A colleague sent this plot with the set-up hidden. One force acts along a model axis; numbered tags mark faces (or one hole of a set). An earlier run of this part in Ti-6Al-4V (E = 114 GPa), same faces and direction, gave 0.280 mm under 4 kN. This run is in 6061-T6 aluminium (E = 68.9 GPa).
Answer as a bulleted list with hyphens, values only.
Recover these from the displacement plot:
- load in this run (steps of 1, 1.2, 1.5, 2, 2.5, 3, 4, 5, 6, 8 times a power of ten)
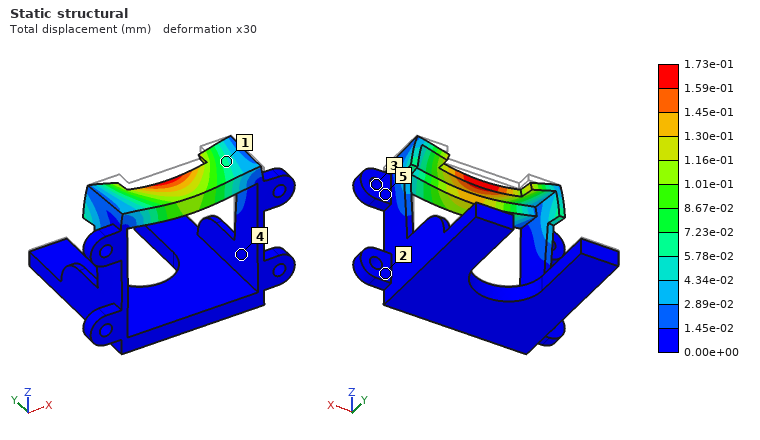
- 1.5 kN
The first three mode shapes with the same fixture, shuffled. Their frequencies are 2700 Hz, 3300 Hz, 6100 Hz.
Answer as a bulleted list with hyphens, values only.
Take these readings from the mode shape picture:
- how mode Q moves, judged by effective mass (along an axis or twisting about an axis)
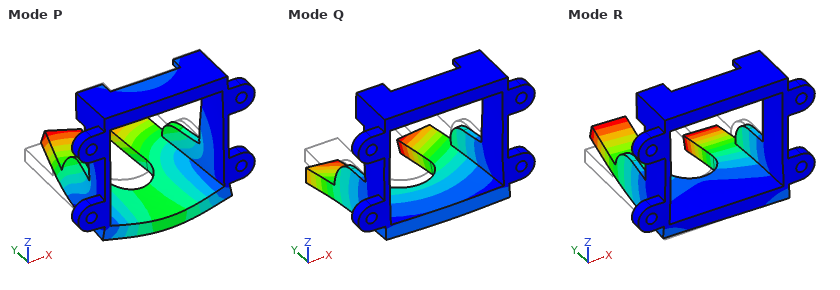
- along Z
